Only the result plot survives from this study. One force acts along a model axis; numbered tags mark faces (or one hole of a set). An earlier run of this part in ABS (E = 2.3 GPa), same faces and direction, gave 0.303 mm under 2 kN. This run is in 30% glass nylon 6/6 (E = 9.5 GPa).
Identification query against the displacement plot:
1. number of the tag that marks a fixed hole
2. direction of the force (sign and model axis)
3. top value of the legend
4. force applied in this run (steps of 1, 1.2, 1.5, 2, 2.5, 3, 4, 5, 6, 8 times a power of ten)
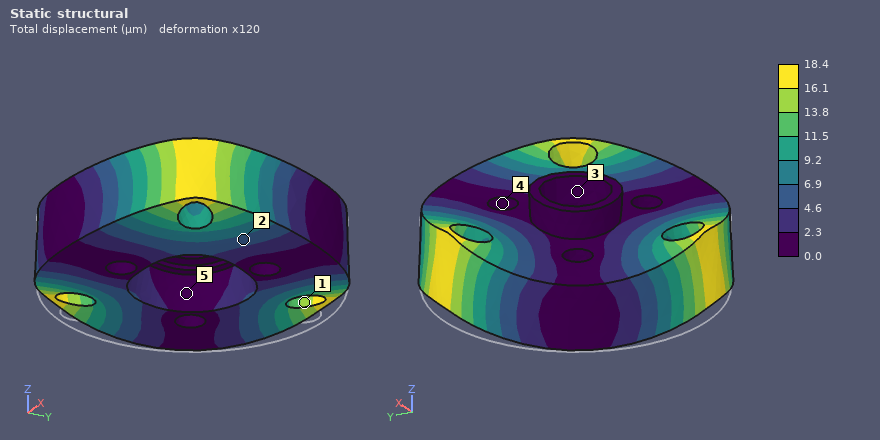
4
+Z
18.4 µm
500 N
